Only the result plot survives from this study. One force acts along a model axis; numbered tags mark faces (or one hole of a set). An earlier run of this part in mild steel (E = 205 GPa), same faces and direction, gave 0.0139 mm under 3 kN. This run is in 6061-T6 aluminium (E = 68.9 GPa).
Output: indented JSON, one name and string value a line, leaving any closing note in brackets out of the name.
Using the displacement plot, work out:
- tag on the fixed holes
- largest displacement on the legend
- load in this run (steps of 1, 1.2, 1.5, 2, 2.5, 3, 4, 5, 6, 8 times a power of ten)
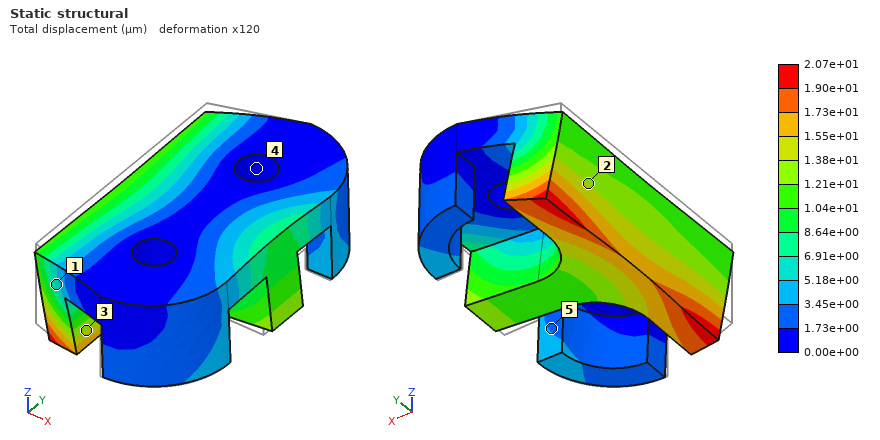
{
  "tag on the fixed holes": "4",
  "largest displacement on the legend": "2.07e+01 µm",
  "load in this run": "1.5 kN"
}
